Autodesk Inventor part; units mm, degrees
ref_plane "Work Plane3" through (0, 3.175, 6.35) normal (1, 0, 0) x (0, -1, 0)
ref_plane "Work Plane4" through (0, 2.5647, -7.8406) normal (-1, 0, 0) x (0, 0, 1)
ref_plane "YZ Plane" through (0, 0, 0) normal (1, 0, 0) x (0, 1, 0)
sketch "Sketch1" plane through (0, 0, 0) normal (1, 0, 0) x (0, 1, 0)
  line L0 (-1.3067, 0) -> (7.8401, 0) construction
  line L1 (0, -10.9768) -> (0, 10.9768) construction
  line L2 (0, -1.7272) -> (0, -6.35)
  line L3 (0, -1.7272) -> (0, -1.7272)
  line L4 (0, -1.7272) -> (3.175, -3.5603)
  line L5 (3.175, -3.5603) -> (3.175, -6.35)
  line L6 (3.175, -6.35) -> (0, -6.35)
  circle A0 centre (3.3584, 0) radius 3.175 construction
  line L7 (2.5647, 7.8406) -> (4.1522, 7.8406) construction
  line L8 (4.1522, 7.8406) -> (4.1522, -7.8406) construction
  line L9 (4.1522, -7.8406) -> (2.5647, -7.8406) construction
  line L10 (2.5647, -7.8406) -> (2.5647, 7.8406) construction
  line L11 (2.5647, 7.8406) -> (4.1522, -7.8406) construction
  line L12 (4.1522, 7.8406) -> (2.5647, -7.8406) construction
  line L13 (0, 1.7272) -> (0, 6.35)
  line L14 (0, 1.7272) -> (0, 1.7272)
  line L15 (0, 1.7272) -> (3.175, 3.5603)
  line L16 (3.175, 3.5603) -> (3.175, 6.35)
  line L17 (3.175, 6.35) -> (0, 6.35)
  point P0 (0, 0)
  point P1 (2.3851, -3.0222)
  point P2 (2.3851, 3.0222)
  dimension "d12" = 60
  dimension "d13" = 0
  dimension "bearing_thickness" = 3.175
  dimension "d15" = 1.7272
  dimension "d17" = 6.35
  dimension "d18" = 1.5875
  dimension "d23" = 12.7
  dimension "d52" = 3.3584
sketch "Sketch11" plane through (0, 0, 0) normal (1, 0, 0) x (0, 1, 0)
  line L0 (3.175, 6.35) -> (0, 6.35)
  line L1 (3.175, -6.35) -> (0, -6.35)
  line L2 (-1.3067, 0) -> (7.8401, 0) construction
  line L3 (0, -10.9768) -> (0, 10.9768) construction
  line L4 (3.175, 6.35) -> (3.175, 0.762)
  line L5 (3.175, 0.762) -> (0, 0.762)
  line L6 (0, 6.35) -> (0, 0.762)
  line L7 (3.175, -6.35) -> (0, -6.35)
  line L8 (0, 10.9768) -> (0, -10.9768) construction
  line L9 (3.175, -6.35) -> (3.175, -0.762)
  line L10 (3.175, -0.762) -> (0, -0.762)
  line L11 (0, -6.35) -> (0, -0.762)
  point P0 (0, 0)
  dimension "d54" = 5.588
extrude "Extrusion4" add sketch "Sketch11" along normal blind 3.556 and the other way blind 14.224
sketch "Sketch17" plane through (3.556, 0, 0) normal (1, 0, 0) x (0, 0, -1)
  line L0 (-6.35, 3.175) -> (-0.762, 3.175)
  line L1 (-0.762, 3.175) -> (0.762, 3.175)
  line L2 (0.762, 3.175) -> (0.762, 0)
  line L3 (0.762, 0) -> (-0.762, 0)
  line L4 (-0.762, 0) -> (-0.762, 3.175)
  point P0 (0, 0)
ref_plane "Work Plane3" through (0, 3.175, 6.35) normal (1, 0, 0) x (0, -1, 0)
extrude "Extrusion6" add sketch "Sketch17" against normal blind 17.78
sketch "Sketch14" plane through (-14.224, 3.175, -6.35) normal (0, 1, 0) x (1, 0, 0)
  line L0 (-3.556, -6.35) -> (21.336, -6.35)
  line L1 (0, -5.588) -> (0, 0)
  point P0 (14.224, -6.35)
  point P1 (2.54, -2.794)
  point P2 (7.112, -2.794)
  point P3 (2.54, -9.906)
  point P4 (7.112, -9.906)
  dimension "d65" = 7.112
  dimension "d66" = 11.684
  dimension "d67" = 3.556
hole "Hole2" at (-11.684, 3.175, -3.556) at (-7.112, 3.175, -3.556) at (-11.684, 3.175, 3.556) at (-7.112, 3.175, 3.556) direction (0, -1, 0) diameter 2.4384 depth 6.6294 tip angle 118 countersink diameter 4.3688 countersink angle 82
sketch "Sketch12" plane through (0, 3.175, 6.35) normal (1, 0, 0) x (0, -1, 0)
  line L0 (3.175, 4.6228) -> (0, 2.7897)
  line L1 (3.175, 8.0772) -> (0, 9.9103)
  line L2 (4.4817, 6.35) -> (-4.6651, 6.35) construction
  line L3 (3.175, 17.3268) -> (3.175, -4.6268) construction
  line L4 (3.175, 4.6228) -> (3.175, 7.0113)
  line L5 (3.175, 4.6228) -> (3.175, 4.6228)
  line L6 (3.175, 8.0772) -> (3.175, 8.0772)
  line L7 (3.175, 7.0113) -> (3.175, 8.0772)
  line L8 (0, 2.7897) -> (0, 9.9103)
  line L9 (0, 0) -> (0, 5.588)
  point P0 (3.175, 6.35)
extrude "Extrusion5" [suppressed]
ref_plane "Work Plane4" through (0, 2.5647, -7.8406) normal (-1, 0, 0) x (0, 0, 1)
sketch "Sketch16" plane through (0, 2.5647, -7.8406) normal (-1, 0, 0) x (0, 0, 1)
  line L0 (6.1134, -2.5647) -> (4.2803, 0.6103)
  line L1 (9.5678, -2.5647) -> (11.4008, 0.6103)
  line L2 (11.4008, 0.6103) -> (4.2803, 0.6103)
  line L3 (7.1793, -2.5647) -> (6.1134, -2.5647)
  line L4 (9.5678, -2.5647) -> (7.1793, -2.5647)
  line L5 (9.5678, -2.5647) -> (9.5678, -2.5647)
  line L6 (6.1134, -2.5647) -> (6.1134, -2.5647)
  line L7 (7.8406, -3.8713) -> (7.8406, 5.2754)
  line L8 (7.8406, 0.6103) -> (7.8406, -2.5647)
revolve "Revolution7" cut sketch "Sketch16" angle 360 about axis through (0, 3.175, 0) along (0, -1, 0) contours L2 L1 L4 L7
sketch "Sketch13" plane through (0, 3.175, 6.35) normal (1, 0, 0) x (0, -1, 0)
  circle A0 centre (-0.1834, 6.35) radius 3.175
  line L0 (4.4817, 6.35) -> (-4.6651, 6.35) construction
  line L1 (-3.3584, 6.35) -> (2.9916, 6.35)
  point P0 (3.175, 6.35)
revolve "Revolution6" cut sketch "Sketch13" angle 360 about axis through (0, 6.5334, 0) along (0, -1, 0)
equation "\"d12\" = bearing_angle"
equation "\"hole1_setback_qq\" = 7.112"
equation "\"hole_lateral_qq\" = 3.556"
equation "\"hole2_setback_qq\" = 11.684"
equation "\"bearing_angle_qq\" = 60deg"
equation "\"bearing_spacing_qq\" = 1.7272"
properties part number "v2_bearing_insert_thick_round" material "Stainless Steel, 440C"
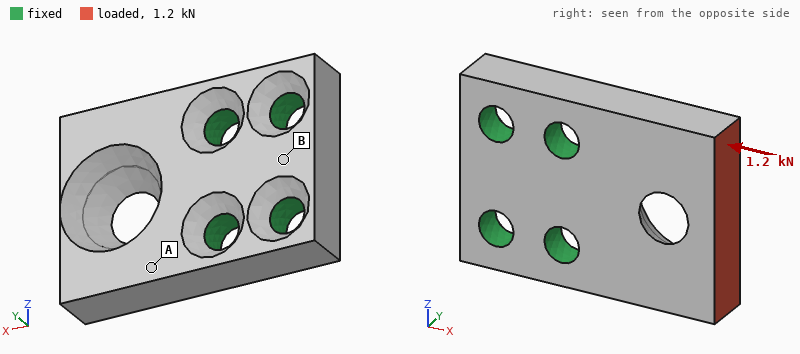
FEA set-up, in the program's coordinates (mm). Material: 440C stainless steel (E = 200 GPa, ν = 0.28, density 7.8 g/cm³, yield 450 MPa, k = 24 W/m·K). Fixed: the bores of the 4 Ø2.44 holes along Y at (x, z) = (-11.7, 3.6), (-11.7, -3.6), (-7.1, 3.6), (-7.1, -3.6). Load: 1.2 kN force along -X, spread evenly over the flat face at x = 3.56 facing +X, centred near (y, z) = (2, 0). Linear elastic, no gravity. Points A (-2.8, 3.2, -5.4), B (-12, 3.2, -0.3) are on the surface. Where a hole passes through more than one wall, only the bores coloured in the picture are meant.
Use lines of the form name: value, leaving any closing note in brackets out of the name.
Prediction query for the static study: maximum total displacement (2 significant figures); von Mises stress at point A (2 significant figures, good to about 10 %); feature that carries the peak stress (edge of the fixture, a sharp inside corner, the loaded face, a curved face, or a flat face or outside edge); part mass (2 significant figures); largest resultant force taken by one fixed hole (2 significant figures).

maximum total displacement: 15 µm
von Mises stress at point A: 52 MPa
feature that carries the peak stress: the loaded face
part mass: 4.4 g
largest resultant force taken by one fixed hole: 520 N
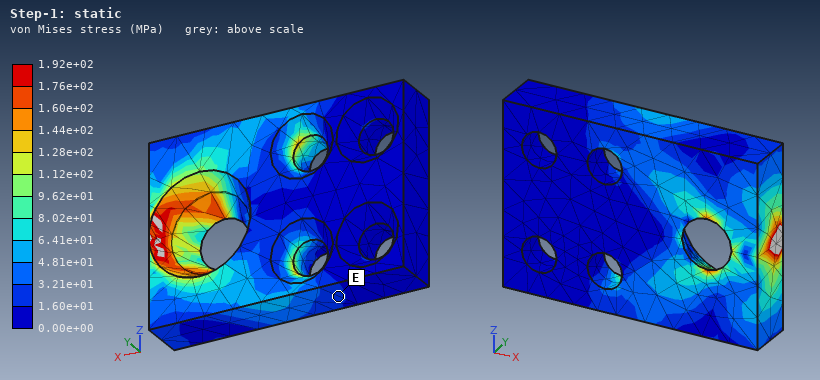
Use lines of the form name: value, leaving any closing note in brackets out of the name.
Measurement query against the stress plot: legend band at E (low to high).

legend band at E: 1.60e+01 to 3.21e+01 MPa
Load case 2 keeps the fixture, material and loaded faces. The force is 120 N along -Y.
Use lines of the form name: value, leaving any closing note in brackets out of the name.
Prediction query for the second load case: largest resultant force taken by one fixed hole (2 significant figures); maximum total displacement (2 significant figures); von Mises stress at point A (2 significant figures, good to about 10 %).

largest resultant force taken by one fixed hole: 100 N
maximum total displacement: 12 µm
von Mises stress at point A: 51 MPa
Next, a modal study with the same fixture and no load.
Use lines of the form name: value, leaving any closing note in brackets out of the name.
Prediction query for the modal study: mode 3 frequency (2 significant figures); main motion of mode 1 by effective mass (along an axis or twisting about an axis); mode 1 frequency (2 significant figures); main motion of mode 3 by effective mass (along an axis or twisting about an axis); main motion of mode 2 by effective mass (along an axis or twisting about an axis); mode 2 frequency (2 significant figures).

mode 3 frequency: 46 kHz
main motion of mode 1 by effective mass: along Y
mode 1 frequency: 21 kHz
main motion of mode 3 by effective mass: along Z
main motion of mode 2 by effective mass: twisting about X
mode 2 frequency: 34 kHz
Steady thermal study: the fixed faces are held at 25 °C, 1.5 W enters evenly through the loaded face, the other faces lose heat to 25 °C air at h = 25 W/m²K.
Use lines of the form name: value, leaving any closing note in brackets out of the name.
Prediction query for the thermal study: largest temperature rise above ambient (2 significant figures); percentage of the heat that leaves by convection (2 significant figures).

largest temperature rise above ambient: 27 K
percentage of the heat that leaves by convection: 5.9 %
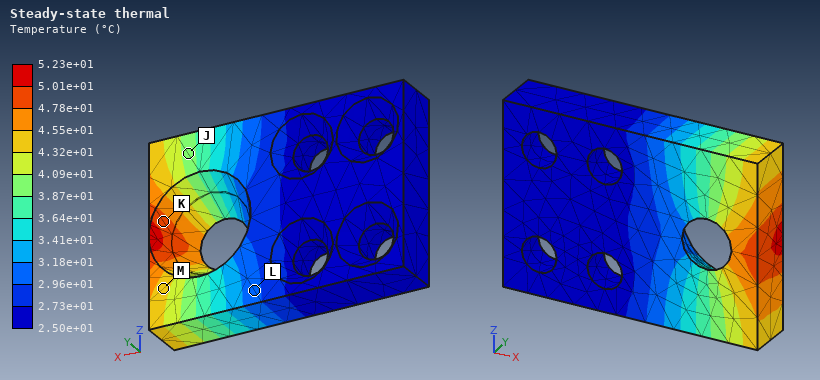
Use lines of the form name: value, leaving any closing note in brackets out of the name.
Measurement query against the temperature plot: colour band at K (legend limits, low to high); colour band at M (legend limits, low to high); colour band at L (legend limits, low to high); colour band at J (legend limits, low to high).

colour band at K: 4.78e+01 to 5.01e+01 °C
colour band at M: 4.32e+01 to 4.55e+01 °C
colour band at L: 2.96e+01 to 3.18e+01 °C
colour band at J: 3.87e+01 to 4.09e+01 °C
